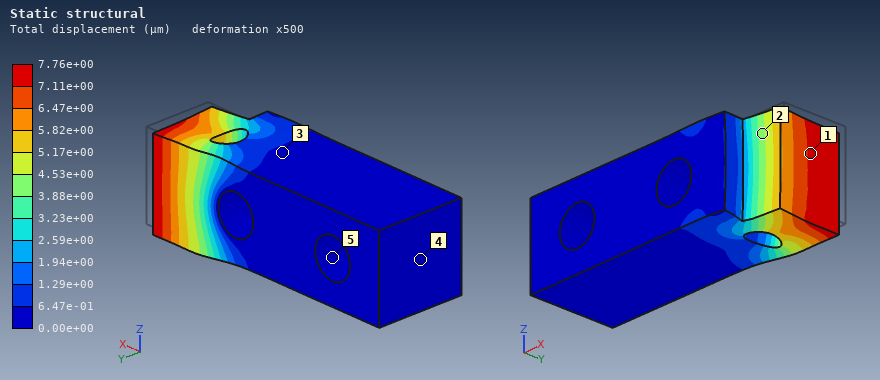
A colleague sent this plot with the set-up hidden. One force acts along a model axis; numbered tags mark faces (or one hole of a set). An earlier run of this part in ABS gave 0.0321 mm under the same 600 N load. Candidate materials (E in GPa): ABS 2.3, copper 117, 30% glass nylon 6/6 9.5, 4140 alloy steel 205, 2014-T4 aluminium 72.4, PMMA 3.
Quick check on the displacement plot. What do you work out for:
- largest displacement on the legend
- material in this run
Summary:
7.76e+00 µm
30% glass nylon 6/6
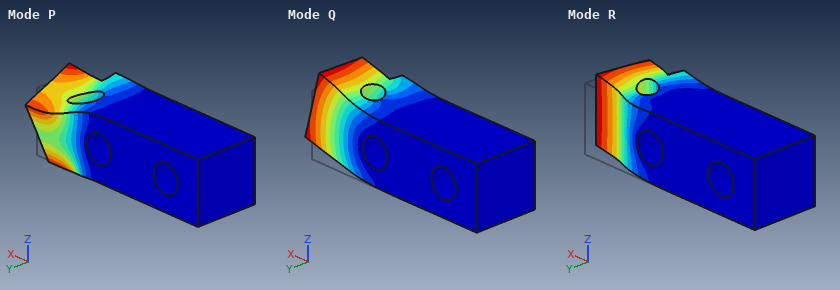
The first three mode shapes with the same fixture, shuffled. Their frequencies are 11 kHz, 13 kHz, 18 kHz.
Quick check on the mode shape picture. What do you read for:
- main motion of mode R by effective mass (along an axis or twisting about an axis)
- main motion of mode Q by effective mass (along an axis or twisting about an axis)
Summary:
along Y
along Z
